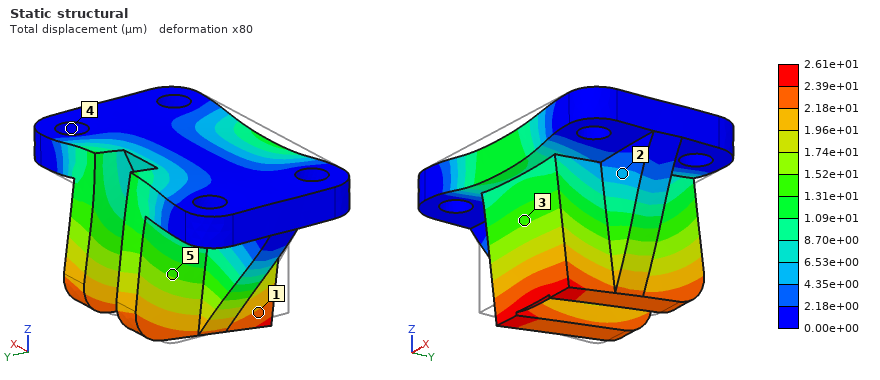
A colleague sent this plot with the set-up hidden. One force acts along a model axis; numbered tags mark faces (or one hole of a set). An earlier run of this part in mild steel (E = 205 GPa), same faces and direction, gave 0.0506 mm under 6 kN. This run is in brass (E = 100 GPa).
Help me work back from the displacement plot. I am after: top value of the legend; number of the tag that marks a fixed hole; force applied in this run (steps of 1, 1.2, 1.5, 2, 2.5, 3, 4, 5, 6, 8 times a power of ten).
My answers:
2.61e+01 µm
4
1.5 kN
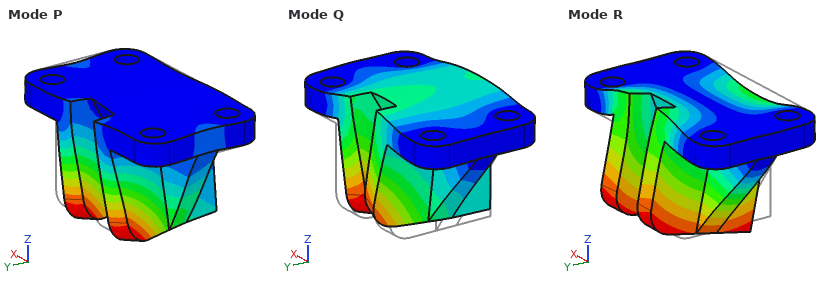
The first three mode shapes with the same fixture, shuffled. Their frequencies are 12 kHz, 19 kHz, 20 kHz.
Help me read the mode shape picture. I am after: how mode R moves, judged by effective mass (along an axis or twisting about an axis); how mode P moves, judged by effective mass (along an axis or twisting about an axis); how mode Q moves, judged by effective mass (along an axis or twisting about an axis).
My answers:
along Y
along X
along Z
